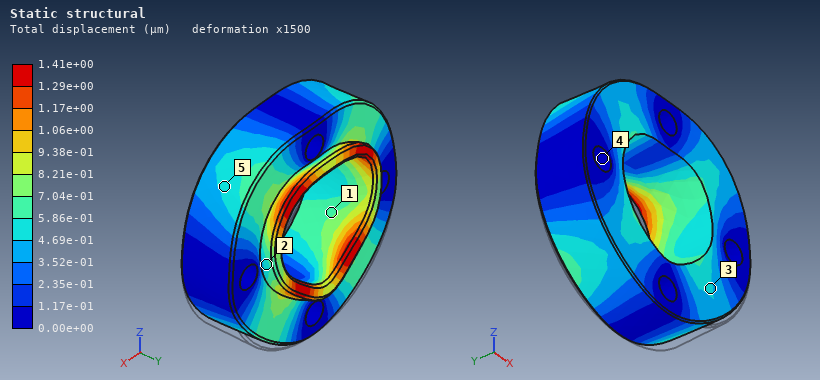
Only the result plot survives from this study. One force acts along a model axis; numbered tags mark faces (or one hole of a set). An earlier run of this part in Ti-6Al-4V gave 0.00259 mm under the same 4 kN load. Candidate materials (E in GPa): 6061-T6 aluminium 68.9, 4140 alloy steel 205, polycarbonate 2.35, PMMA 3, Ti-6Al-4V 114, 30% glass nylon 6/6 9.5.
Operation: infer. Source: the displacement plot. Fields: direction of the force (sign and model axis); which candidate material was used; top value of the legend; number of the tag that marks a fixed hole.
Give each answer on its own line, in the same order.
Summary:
+Z
4140 alloy steel
1.41e+00 µm
4
